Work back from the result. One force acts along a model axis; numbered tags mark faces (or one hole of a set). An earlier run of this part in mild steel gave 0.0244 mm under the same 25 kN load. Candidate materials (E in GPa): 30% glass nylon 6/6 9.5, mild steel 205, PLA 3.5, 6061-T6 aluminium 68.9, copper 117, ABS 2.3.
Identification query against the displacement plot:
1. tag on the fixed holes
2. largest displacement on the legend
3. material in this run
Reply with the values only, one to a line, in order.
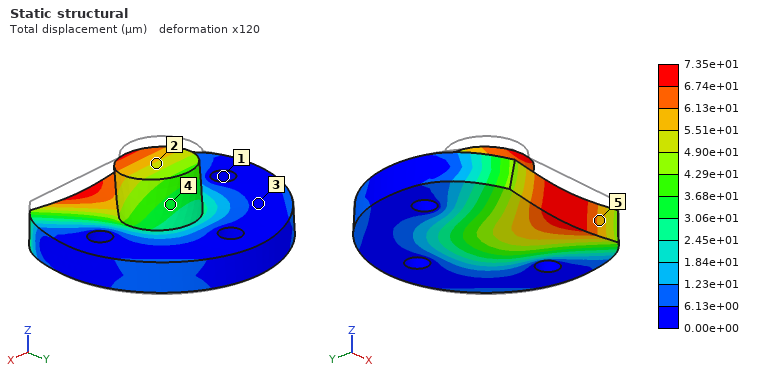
1
7.35e+01 µm
6061-T6 aluminium
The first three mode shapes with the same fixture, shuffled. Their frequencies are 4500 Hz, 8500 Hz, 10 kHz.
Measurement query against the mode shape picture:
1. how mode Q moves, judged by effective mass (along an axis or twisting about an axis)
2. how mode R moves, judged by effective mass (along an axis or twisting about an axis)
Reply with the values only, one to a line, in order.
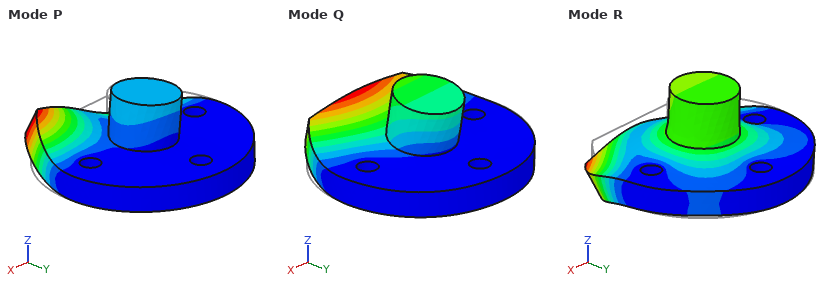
along Z
along Z
